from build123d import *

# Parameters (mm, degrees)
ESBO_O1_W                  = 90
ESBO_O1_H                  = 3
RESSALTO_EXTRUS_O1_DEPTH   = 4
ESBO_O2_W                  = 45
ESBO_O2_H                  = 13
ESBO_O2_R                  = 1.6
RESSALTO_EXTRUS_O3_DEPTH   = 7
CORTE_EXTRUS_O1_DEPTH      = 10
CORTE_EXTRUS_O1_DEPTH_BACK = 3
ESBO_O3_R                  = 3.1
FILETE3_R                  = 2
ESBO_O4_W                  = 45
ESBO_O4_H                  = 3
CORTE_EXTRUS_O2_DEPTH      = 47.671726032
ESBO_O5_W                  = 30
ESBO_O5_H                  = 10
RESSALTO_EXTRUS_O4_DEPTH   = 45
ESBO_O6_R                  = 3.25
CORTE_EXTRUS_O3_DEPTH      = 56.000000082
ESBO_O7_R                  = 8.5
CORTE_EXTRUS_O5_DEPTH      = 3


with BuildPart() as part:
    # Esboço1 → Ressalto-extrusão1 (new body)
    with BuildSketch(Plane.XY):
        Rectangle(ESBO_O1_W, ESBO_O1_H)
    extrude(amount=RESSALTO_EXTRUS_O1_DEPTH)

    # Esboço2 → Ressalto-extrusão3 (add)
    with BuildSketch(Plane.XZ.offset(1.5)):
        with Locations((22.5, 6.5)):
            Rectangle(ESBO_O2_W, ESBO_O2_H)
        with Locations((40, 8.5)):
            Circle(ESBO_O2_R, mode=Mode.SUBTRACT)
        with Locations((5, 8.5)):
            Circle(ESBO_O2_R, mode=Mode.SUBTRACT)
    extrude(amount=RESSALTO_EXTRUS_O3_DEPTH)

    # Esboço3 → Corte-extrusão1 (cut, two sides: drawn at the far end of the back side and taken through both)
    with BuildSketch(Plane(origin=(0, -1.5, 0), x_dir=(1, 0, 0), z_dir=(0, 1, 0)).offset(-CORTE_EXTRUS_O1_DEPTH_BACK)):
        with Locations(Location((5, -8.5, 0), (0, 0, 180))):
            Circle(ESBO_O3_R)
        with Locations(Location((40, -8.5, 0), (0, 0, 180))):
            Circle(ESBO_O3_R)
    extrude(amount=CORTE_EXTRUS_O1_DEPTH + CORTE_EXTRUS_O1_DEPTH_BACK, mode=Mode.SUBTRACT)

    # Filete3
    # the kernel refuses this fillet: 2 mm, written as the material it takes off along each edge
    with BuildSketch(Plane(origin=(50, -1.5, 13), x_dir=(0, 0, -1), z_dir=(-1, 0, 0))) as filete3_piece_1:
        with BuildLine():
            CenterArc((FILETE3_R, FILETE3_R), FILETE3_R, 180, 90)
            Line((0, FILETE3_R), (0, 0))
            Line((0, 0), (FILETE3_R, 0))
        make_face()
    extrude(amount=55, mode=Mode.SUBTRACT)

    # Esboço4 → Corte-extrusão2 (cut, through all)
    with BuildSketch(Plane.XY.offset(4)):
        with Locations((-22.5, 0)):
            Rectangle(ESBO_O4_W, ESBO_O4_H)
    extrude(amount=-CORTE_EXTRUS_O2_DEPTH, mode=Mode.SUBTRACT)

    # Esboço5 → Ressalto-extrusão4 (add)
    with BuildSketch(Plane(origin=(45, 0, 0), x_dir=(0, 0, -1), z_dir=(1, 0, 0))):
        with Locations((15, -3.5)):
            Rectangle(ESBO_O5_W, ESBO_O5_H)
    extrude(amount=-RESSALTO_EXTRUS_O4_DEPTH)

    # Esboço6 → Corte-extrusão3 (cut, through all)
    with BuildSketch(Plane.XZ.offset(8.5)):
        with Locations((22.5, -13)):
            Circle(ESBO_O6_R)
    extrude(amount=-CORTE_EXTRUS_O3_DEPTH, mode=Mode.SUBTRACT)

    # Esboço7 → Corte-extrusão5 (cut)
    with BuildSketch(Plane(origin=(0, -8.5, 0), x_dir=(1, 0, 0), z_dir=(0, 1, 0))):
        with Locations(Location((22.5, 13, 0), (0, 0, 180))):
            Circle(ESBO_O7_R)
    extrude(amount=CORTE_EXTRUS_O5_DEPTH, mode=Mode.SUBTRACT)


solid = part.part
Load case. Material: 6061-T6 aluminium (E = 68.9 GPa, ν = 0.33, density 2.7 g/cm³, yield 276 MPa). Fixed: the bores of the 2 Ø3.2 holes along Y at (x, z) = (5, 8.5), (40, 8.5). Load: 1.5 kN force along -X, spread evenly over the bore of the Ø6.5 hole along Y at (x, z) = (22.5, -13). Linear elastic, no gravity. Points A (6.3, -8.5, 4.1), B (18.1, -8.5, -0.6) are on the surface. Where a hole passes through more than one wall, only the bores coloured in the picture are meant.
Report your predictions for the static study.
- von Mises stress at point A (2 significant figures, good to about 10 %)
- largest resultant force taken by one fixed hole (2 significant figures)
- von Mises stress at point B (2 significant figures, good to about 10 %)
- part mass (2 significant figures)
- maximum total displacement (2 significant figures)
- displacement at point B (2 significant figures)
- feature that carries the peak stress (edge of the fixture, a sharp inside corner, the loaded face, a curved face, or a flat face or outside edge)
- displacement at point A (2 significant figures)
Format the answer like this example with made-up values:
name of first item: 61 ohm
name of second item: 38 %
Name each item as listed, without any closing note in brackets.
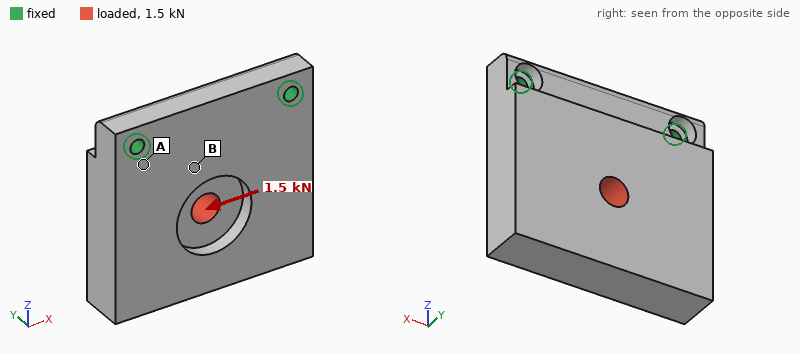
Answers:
von Mises stress at point A: 20 MPa
largest resultant force taken by one fixed hole: 1.2 kN
von Mises stress at point B: 9.2 MPa
part mass: 46 g
maximum total displacement: 11 µm
displacement at point B: 3.6 µm
feature that carries the peak stress: edge of the fixture
displacement at point A: 1.8 µm
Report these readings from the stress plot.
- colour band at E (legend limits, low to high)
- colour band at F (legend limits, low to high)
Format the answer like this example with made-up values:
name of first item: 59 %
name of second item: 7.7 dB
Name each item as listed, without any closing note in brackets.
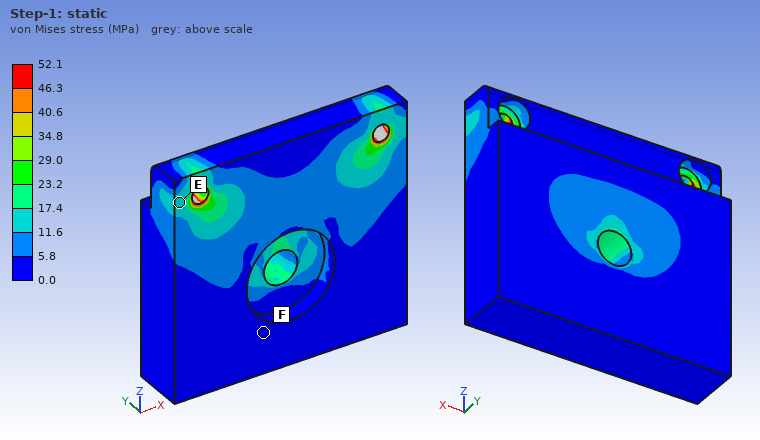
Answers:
colour band at E: 11.6 to 17.4 MPa
colour band at F: 0.0 to 5.8 MPa
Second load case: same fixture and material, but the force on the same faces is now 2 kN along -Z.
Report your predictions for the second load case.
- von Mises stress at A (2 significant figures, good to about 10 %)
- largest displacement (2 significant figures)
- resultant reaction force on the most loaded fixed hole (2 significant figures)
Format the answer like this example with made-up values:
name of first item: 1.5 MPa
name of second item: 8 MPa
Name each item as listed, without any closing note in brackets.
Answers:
von Mises stress at A: 22 MPa
largest displacement: 95 µm
resultant reaction force on the most loaded fixed hole: 1.0 kN
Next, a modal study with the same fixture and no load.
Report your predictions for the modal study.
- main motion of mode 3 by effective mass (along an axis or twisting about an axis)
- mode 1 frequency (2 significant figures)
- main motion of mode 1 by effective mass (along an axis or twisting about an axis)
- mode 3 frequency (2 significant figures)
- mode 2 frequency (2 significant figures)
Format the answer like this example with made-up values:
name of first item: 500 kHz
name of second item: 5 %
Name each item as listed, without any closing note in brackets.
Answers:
main motion of mode 3 by effective mass: along X
mode 1 frequency: 2000 Hz
main motion of mode 1 by effective mass: along Y
mode 3 frequency: 11 kHz
mode 2 frequency: 7300 Hz
